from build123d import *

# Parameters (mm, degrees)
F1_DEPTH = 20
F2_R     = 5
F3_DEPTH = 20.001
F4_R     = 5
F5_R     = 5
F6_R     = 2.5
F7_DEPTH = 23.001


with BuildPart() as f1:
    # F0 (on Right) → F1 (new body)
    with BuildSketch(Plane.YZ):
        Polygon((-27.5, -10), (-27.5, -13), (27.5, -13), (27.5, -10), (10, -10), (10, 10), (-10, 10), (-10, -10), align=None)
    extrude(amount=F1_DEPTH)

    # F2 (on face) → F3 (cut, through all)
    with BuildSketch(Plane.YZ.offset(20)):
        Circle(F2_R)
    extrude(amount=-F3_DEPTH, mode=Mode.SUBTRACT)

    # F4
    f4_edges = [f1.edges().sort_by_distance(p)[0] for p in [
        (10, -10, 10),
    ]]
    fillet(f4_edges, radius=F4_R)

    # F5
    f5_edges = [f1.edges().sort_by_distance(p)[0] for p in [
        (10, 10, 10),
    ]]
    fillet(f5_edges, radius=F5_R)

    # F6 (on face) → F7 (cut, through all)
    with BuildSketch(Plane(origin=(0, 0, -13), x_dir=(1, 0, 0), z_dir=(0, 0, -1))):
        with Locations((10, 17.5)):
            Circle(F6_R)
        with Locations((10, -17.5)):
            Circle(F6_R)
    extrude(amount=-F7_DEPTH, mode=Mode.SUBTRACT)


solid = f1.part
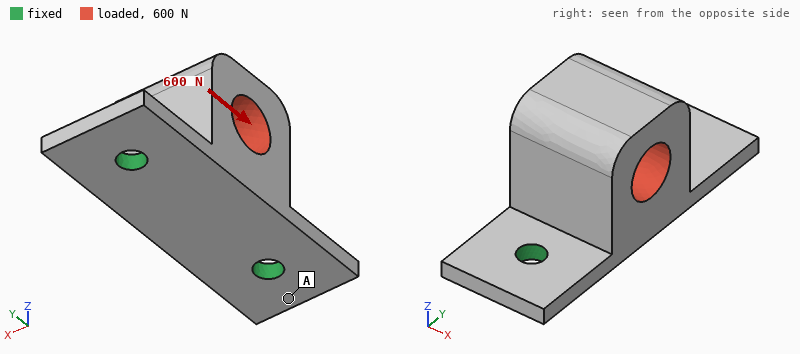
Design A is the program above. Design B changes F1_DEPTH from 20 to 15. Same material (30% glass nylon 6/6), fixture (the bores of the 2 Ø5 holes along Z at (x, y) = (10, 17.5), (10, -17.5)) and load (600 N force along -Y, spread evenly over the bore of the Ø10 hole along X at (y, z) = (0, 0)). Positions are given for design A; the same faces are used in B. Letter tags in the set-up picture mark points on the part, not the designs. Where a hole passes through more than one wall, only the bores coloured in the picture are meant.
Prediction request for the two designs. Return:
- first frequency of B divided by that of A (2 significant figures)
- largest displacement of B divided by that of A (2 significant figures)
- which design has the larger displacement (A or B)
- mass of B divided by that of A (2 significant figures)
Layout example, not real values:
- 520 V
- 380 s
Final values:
- 0.98
- 1.2
- B
- 0.75
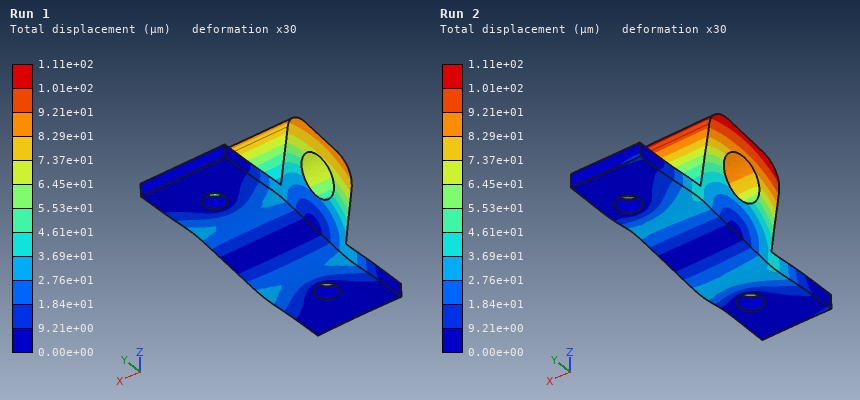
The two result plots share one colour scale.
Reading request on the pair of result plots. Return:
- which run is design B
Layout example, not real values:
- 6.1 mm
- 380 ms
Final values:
- Run 2
